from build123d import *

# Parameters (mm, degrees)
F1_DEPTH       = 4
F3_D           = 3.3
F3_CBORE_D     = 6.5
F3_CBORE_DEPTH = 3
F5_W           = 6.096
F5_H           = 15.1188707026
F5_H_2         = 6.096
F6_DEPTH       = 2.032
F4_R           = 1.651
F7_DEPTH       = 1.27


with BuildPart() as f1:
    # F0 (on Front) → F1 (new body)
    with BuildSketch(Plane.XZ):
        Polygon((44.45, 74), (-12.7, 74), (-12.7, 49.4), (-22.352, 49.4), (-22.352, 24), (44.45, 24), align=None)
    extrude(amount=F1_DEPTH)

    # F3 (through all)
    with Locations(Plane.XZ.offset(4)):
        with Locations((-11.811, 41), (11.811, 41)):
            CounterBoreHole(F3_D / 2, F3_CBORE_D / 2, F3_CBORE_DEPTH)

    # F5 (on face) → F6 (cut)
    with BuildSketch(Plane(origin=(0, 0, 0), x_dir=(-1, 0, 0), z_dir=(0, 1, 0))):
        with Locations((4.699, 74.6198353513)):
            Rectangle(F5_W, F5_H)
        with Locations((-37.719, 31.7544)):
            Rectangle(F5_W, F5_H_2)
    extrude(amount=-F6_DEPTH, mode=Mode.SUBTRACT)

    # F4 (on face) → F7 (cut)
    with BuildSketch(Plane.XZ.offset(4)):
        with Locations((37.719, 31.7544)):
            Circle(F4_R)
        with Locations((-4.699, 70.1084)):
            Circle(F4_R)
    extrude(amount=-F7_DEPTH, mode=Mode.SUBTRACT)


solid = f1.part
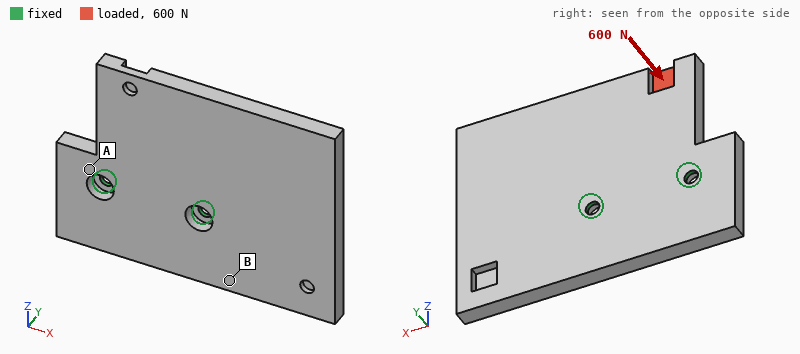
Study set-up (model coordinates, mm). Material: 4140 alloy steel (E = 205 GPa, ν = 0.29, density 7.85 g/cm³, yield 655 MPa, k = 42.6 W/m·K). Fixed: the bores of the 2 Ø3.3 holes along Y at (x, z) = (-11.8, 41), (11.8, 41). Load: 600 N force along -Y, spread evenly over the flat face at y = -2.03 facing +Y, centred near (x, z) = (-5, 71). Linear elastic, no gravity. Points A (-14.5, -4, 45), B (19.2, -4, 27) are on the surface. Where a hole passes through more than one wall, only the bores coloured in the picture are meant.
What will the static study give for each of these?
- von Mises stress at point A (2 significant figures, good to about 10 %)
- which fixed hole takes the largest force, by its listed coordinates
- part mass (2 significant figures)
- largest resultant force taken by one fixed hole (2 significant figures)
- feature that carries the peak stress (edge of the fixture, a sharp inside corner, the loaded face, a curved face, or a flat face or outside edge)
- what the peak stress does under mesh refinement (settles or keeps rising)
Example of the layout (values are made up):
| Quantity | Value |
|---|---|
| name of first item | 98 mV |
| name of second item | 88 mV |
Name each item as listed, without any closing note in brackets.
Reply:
| Quantity | Value |
|---|---|
| von Mises stress at point A | 260 MPa |
| which fixed hole takes the largest force, by its listed coordinates | (-11.8, 41) |
| part mass | 94 g |
| largest resultant force taken by one fixed hole | 570 N |
| feature that carries the peak stress | edge of the fixture |
| what the peak stress does under mesh refinement | keeps rising |
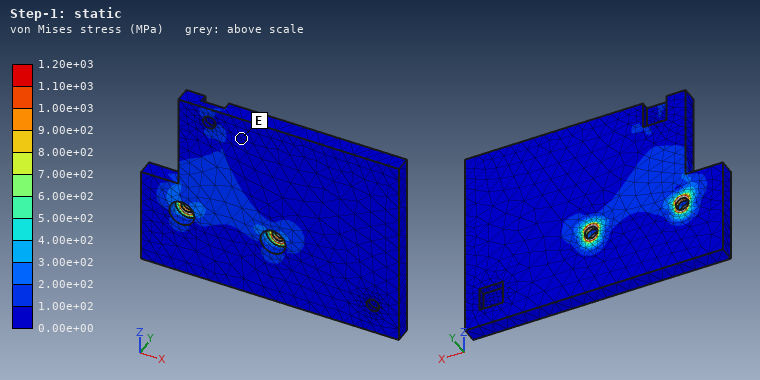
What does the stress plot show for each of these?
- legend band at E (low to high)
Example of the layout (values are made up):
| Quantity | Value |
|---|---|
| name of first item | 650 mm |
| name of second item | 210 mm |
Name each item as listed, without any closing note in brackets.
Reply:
| Quantity | Value |
|---|---|
| legend band at E | 0.00e+00 to 1.00e+02 MPa |
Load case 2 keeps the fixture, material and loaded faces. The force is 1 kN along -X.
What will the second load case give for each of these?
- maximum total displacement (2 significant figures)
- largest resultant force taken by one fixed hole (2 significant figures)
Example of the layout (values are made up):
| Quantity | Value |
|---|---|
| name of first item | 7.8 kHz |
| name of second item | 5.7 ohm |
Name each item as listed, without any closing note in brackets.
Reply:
| Quantity | Value |
|---|---|
| maximum total displacement | 19 µm |
| largest resultant force taken by one fixed hole | 1.3 kN |
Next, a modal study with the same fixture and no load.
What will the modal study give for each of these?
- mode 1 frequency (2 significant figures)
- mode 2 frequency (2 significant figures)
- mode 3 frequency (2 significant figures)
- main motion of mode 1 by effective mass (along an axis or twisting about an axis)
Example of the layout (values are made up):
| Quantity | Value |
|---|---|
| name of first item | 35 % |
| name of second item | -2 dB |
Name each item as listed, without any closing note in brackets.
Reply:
| Quantity | Value |
|---|---|
| mode 1 frequency | 1100 Hz |
| mode 2 frequency | 2200 Hz |
| mode 3 frequency | 4400 Hz |
| main motion of mode 1 by effective mass | along Y |
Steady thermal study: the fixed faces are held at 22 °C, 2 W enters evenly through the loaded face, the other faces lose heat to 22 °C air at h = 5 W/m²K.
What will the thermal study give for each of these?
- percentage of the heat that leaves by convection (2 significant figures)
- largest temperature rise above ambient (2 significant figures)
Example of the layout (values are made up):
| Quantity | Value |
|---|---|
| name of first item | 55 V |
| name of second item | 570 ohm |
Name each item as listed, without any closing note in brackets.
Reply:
| Quantity | Value |
|---|---|
| percentage of the heat that leaves by convection | 9.9 % |
| largest temperature rise above ambient | 19 K |
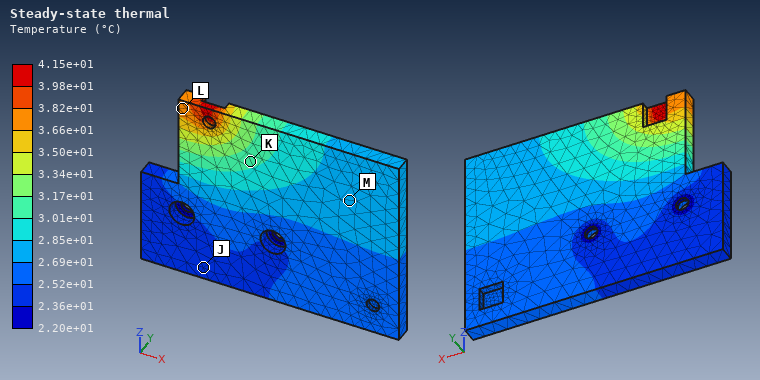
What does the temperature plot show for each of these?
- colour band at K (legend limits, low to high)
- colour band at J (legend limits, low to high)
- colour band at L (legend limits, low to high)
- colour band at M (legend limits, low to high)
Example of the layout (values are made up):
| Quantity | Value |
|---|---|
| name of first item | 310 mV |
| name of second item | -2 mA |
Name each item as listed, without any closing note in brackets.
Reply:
| Quantity | Value |
|---|---|
| colour band at K | 3.01e+01 to 3.17e+01 °C |
| colour band at J | 2.36e+01 to 2.52e+01 °C |
| colour band at L | 3.66e+01 to 3.82e+01 °C |
| colour band at M | 2.69e+01 to 2.85e+01 °C |
